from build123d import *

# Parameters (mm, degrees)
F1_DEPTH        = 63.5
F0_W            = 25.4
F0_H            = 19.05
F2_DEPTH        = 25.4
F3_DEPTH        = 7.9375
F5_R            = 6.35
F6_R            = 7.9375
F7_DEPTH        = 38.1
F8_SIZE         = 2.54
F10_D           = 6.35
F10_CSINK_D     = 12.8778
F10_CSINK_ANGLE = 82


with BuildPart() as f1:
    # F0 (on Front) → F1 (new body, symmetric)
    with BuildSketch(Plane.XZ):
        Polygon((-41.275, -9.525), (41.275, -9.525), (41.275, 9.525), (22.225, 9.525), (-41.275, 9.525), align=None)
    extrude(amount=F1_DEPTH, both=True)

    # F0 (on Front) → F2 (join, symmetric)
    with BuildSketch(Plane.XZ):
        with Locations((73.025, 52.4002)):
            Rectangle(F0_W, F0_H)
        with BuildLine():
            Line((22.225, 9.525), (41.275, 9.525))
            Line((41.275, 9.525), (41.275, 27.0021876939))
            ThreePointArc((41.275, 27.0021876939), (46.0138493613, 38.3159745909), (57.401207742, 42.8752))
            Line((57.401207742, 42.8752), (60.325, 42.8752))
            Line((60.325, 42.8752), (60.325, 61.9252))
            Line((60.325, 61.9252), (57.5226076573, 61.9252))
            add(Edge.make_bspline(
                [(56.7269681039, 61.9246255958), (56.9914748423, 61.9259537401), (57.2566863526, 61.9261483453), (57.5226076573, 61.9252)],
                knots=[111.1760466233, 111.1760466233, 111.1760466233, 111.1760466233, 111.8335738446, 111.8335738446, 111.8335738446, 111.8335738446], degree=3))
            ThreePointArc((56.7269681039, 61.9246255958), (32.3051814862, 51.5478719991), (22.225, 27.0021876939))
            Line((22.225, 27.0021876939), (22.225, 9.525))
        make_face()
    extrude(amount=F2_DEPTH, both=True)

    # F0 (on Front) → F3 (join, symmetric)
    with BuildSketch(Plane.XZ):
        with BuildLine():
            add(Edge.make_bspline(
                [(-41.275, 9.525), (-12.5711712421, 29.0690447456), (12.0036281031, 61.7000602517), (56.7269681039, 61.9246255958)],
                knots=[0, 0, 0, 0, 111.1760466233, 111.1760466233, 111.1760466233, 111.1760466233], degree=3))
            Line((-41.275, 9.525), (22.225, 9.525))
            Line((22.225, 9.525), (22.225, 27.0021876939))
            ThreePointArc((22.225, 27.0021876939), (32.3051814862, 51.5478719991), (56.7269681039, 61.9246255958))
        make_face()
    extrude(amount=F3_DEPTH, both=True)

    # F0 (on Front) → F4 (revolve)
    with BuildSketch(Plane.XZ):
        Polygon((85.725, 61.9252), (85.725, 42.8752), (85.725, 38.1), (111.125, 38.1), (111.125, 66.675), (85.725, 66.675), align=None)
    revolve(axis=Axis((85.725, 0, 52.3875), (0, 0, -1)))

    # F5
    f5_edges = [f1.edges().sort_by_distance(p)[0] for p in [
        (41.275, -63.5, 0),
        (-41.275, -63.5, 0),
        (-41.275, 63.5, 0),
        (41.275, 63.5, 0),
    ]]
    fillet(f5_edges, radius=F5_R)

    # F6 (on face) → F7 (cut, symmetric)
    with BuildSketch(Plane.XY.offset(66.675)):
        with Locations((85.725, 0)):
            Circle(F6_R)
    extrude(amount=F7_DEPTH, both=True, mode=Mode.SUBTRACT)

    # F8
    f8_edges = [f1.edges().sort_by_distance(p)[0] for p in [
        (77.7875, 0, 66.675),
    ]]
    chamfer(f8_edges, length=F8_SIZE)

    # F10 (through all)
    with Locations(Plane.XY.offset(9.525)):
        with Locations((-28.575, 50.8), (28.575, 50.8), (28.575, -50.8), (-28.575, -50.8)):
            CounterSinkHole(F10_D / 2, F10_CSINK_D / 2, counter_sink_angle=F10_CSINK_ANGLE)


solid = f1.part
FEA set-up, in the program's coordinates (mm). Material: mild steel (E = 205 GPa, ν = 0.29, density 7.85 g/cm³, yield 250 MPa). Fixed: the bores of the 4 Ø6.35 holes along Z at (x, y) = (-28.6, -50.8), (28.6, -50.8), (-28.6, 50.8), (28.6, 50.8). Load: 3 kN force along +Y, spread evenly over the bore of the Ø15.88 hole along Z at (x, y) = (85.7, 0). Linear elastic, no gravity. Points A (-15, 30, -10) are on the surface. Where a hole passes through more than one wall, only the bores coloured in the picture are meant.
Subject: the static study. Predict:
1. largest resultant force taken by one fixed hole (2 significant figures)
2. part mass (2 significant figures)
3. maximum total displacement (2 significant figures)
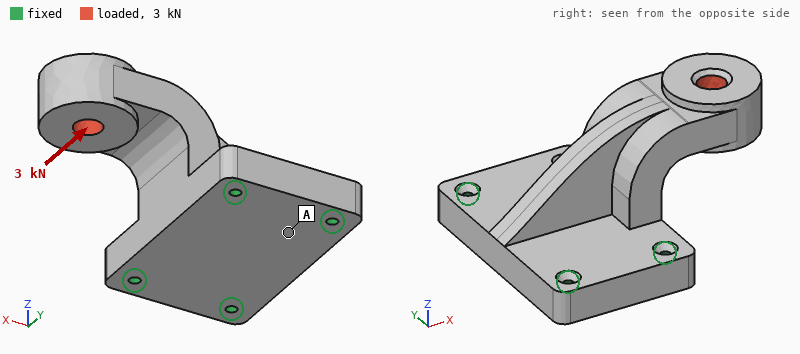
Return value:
2.4 kN
2.7 kg
54 µm
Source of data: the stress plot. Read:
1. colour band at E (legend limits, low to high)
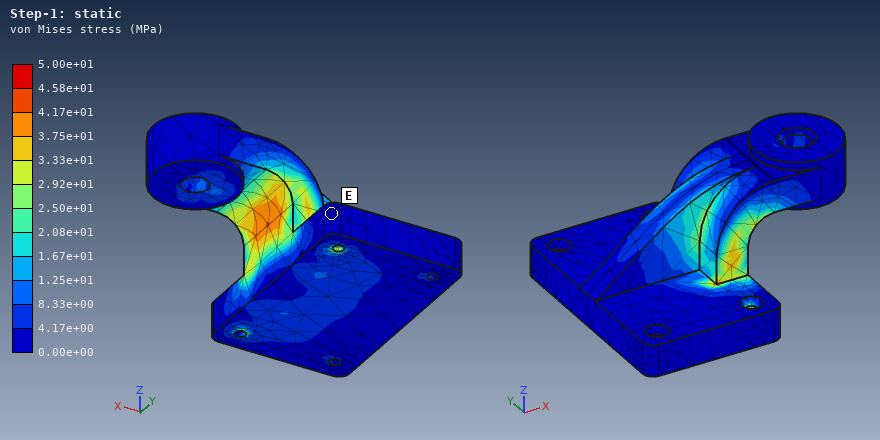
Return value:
0.00e+00 to 4.17e+00 MPa
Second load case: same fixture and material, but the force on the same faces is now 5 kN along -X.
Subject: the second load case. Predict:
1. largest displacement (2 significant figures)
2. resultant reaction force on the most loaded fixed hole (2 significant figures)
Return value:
42 µm
2.8 kN
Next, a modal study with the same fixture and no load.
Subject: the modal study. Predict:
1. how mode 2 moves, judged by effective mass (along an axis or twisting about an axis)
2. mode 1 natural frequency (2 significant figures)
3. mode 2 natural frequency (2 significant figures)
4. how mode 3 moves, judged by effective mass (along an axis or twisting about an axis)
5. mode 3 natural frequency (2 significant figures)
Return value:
along Y
1600 Hz
1900 Hz
along X
4000 Hz
